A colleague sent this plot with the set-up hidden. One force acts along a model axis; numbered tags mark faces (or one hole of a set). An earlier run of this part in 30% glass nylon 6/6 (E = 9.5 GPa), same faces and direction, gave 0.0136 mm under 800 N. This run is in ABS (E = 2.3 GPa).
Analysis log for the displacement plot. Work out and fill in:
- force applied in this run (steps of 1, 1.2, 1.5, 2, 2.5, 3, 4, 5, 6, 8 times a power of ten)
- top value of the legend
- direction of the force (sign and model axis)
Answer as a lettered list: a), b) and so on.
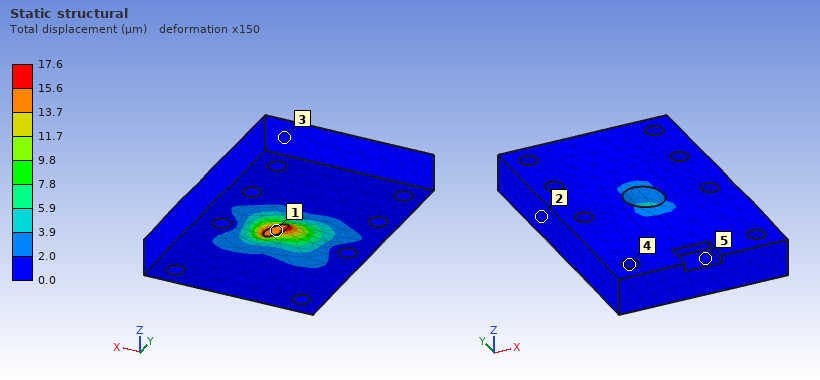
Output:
a) 250 N
b) 17.6 µm
c) +X
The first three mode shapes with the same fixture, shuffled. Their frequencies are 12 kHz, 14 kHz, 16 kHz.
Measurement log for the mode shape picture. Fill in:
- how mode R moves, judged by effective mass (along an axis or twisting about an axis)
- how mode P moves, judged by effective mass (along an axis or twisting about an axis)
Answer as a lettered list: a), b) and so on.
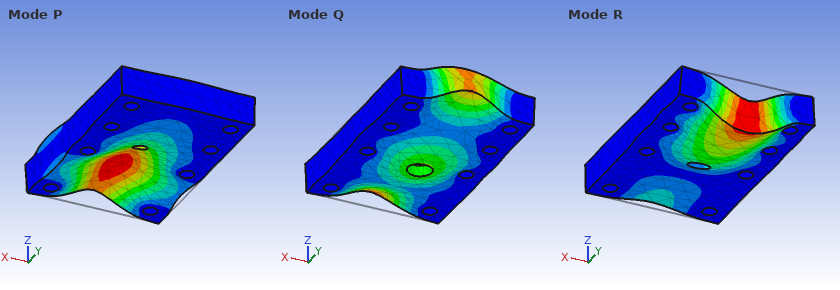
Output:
a) along Z
b) along Z
